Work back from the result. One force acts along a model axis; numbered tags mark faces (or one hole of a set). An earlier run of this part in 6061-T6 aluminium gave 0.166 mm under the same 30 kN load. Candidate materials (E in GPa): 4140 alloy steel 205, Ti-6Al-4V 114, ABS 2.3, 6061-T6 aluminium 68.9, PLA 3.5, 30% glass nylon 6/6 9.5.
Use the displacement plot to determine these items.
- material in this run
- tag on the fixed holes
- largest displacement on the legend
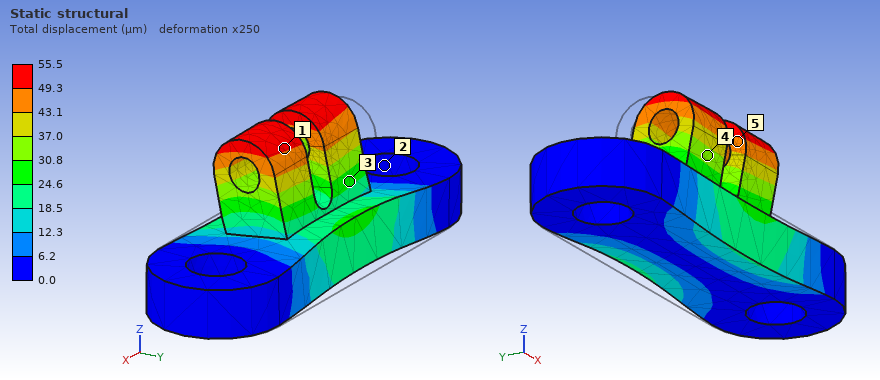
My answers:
4140 alloy steel
2
55.5 µm
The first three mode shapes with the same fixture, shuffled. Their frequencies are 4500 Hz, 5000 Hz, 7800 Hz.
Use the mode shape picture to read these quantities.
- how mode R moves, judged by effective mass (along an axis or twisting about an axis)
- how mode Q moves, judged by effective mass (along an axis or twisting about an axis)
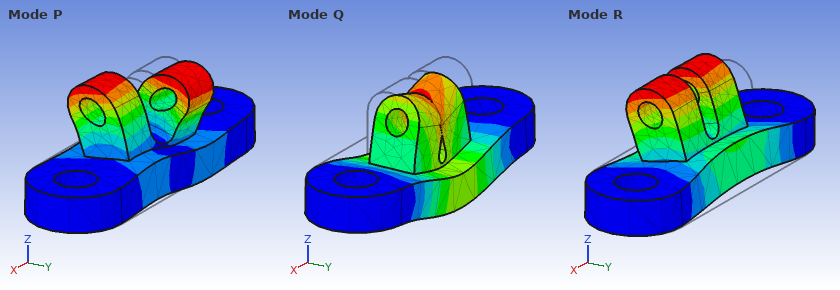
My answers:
along Y
along Z
